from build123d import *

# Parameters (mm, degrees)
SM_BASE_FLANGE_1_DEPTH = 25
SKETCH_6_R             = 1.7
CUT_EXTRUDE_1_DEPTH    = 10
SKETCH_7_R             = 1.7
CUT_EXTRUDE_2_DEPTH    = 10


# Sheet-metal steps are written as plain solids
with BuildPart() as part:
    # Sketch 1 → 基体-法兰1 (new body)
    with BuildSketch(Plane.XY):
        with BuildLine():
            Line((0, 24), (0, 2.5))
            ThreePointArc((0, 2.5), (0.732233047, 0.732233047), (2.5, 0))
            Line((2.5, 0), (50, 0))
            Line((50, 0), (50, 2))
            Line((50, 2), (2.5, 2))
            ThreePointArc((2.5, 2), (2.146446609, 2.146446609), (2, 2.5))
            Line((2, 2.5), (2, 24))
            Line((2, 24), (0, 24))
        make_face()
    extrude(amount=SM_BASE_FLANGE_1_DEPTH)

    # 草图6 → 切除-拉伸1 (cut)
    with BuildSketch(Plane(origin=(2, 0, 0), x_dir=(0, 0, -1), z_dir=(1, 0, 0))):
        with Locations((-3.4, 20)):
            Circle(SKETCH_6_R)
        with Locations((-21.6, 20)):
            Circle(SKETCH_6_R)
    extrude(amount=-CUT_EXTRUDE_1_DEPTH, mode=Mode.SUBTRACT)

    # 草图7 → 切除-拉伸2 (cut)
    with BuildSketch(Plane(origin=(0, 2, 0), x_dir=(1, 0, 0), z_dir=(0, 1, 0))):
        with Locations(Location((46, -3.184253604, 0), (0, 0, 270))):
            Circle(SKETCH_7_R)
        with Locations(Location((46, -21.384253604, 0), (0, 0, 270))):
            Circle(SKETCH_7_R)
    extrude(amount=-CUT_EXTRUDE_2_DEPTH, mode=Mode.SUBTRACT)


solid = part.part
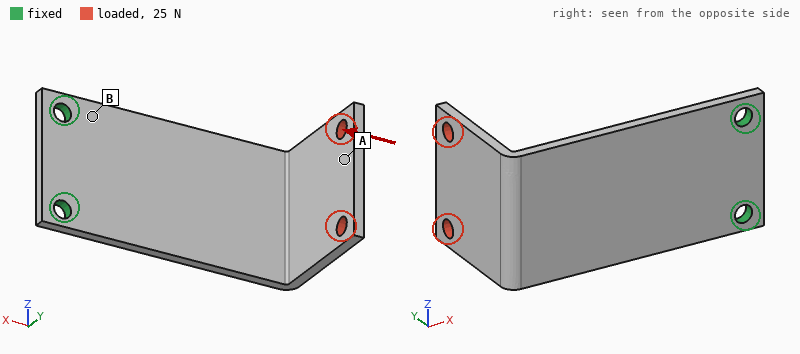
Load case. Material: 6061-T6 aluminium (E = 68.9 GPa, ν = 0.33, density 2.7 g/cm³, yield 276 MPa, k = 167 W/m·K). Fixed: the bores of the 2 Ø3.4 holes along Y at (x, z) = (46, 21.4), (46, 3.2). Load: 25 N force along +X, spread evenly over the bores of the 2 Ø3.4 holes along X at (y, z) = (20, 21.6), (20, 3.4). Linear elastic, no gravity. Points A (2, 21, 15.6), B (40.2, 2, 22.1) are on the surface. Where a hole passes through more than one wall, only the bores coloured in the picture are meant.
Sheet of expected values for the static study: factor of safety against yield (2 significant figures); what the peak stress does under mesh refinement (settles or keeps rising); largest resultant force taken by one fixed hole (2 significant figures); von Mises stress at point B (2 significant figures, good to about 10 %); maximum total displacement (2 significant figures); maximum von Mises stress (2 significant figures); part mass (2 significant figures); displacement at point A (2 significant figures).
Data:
4.6
settles
13 N
31 MPa
0.63 mm
59 MPa
9.4 g
0.56 mm
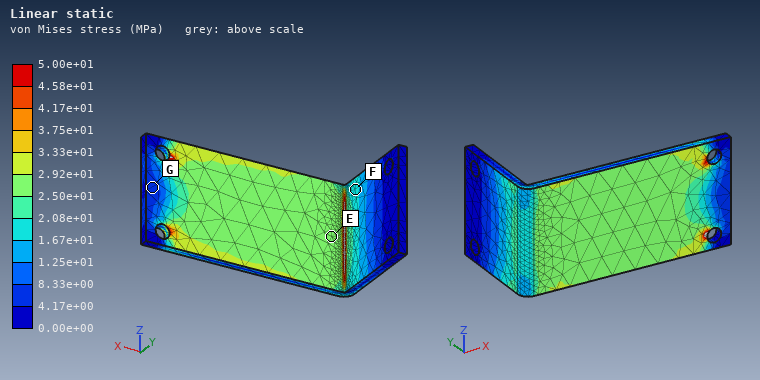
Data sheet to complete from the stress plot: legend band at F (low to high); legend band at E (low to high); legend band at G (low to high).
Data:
1.67e+01 to 2.08e+01 MPa
2.50e+01 to 2.92e+01 MPa
4.17e+00 to 8.33e+00 MPa
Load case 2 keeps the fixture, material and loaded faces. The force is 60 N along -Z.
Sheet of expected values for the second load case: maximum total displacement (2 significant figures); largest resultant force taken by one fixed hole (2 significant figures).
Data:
0.64 mm
150 N
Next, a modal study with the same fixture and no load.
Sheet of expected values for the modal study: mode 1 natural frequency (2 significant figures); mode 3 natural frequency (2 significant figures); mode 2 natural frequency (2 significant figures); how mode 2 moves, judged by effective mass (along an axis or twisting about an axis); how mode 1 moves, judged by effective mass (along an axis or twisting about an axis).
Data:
450 Hz
1800 Hz
1200 Hz
along Z
along Y
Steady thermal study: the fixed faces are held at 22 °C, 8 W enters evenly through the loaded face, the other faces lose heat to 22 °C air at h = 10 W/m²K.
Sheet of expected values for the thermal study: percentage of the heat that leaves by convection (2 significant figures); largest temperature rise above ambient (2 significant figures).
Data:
13 %
59 K
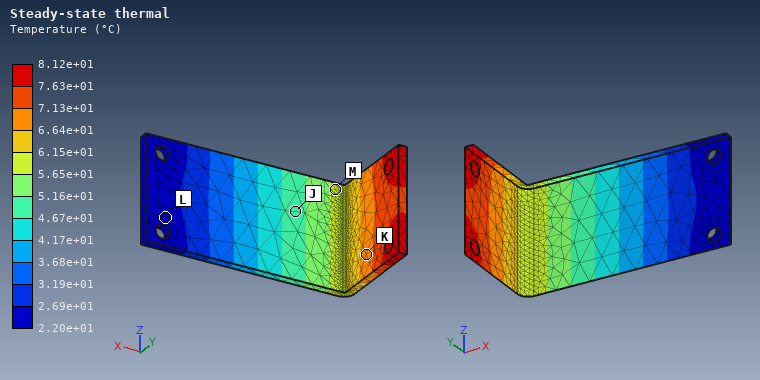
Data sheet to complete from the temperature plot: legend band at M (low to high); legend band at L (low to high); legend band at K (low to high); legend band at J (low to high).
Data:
5.65e+01 to 6.15e+01 °C
2.20e+01 to 2.69e+01 °C
6.64e+01 to 7.13e+01 °C
4.67e+01 to 5.16e+01 °C
